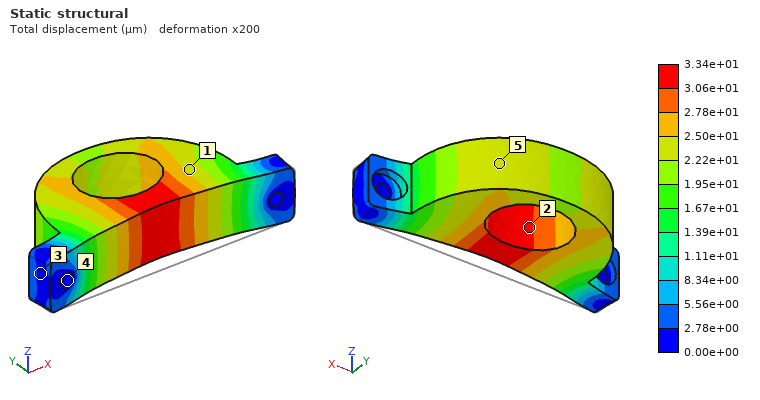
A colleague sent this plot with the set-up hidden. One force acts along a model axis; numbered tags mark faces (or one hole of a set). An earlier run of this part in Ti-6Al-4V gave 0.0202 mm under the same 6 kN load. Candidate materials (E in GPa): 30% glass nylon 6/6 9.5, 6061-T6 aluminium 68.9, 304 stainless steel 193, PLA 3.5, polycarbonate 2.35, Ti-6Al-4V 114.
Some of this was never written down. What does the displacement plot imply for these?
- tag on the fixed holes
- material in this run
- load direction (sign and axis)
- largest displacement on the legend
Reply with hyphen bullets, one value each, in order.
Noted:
- 4
- 6061-T6 aluminium
- +Y
- 3.34e+01 µm
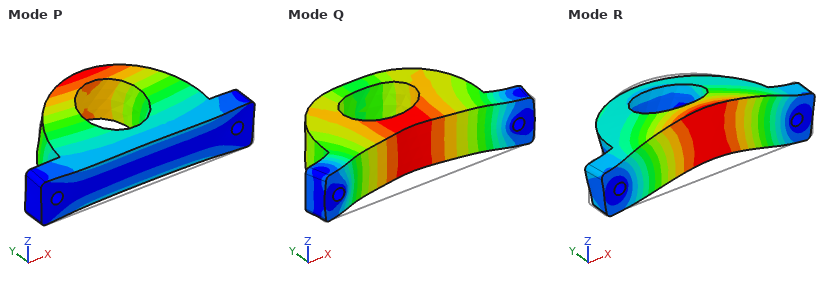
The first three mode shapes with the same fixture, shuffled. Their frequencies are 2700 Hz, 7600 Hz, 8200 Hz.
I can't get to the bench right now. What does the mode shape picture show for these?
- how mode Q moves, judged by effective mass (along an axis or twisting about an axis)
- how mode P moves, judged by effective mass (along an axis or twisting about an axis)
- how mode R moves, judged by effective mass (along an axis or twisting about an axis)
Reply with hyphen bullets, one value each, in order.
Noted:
- along Y
- along Z
- along Z
